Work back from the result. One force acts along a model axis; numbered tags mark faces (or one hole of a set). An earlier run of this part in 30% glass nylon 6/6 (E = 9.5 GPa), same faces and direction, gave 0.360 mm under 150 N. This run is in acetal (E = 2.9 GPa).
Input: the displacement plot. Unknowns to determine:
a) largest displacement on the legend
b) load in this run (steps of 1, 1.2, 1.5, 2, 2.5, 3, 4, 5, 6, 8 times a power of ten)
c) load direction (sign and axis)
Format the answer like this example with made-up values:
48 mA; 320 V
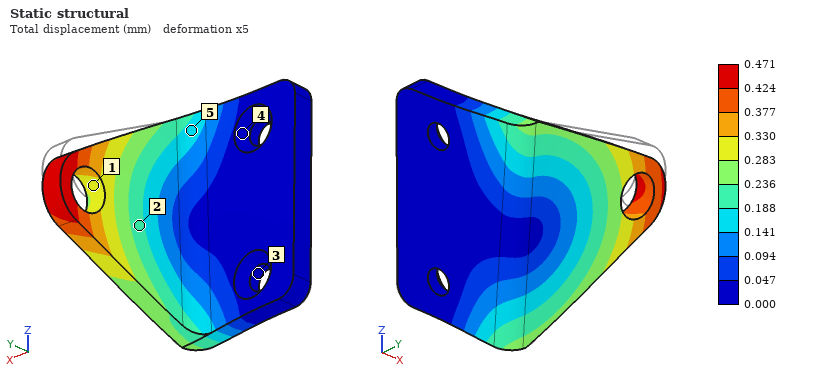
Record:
0.471 mm; 60 N; -Z
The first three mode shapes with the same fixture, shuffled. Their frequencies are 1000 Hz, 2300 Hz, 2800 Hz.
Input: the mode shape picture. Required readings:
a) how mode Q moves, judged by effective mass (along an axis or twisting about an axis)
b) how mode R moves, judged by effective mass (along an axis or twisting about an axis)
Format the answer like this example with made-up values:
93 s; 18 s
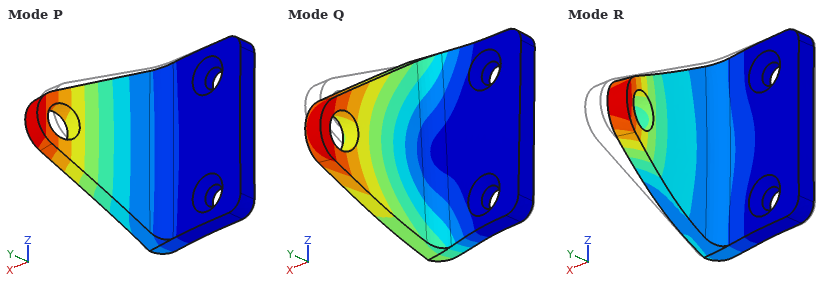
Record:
along Z; along Y
